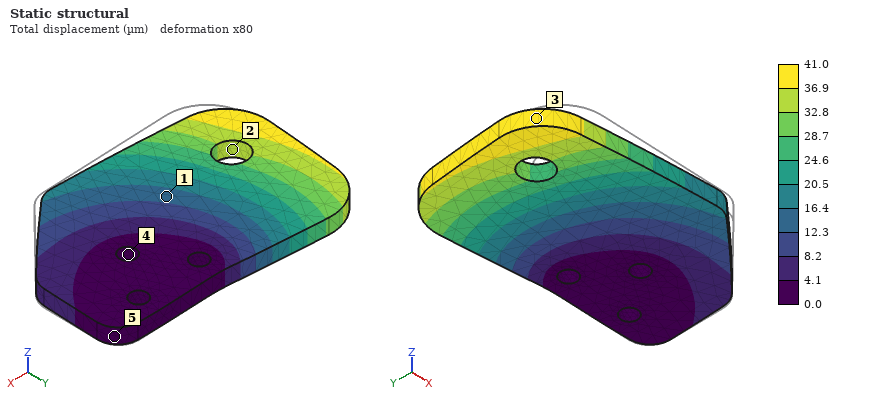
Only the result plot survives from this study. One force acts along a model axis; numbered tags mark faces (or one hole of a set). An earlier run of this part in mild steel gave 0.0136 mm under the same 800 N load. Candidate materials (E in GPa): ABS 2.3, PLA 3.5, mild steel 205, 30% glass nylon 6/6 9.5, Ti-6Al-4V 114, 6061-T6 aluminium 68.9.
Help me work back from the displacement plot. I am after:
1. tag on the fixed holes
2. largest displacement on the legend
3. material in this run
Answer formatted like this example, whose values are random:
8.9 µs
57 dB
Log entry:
4
41.0 µm
6061-T6 aluminium
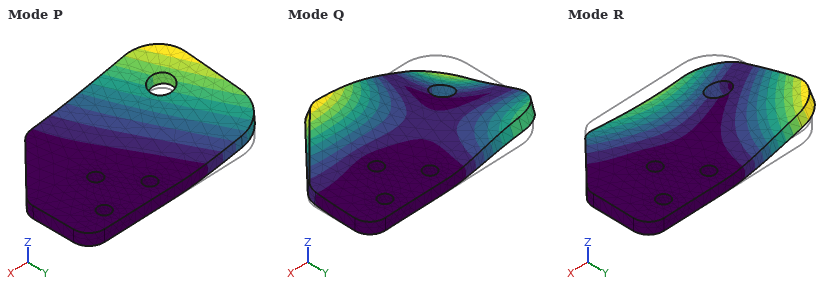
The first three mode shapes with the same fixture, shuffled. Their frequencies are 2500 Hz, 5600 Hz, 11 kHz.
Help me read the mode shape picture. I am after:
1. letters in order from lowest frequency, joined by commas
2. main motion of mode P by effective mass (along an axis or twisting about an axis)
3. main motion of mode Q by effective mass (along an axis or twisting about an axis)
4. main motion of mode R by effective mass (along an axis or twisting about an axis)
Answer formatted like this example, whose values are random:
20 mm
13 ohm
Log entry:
P, R, Q
along Z
along Z
twisting about X
